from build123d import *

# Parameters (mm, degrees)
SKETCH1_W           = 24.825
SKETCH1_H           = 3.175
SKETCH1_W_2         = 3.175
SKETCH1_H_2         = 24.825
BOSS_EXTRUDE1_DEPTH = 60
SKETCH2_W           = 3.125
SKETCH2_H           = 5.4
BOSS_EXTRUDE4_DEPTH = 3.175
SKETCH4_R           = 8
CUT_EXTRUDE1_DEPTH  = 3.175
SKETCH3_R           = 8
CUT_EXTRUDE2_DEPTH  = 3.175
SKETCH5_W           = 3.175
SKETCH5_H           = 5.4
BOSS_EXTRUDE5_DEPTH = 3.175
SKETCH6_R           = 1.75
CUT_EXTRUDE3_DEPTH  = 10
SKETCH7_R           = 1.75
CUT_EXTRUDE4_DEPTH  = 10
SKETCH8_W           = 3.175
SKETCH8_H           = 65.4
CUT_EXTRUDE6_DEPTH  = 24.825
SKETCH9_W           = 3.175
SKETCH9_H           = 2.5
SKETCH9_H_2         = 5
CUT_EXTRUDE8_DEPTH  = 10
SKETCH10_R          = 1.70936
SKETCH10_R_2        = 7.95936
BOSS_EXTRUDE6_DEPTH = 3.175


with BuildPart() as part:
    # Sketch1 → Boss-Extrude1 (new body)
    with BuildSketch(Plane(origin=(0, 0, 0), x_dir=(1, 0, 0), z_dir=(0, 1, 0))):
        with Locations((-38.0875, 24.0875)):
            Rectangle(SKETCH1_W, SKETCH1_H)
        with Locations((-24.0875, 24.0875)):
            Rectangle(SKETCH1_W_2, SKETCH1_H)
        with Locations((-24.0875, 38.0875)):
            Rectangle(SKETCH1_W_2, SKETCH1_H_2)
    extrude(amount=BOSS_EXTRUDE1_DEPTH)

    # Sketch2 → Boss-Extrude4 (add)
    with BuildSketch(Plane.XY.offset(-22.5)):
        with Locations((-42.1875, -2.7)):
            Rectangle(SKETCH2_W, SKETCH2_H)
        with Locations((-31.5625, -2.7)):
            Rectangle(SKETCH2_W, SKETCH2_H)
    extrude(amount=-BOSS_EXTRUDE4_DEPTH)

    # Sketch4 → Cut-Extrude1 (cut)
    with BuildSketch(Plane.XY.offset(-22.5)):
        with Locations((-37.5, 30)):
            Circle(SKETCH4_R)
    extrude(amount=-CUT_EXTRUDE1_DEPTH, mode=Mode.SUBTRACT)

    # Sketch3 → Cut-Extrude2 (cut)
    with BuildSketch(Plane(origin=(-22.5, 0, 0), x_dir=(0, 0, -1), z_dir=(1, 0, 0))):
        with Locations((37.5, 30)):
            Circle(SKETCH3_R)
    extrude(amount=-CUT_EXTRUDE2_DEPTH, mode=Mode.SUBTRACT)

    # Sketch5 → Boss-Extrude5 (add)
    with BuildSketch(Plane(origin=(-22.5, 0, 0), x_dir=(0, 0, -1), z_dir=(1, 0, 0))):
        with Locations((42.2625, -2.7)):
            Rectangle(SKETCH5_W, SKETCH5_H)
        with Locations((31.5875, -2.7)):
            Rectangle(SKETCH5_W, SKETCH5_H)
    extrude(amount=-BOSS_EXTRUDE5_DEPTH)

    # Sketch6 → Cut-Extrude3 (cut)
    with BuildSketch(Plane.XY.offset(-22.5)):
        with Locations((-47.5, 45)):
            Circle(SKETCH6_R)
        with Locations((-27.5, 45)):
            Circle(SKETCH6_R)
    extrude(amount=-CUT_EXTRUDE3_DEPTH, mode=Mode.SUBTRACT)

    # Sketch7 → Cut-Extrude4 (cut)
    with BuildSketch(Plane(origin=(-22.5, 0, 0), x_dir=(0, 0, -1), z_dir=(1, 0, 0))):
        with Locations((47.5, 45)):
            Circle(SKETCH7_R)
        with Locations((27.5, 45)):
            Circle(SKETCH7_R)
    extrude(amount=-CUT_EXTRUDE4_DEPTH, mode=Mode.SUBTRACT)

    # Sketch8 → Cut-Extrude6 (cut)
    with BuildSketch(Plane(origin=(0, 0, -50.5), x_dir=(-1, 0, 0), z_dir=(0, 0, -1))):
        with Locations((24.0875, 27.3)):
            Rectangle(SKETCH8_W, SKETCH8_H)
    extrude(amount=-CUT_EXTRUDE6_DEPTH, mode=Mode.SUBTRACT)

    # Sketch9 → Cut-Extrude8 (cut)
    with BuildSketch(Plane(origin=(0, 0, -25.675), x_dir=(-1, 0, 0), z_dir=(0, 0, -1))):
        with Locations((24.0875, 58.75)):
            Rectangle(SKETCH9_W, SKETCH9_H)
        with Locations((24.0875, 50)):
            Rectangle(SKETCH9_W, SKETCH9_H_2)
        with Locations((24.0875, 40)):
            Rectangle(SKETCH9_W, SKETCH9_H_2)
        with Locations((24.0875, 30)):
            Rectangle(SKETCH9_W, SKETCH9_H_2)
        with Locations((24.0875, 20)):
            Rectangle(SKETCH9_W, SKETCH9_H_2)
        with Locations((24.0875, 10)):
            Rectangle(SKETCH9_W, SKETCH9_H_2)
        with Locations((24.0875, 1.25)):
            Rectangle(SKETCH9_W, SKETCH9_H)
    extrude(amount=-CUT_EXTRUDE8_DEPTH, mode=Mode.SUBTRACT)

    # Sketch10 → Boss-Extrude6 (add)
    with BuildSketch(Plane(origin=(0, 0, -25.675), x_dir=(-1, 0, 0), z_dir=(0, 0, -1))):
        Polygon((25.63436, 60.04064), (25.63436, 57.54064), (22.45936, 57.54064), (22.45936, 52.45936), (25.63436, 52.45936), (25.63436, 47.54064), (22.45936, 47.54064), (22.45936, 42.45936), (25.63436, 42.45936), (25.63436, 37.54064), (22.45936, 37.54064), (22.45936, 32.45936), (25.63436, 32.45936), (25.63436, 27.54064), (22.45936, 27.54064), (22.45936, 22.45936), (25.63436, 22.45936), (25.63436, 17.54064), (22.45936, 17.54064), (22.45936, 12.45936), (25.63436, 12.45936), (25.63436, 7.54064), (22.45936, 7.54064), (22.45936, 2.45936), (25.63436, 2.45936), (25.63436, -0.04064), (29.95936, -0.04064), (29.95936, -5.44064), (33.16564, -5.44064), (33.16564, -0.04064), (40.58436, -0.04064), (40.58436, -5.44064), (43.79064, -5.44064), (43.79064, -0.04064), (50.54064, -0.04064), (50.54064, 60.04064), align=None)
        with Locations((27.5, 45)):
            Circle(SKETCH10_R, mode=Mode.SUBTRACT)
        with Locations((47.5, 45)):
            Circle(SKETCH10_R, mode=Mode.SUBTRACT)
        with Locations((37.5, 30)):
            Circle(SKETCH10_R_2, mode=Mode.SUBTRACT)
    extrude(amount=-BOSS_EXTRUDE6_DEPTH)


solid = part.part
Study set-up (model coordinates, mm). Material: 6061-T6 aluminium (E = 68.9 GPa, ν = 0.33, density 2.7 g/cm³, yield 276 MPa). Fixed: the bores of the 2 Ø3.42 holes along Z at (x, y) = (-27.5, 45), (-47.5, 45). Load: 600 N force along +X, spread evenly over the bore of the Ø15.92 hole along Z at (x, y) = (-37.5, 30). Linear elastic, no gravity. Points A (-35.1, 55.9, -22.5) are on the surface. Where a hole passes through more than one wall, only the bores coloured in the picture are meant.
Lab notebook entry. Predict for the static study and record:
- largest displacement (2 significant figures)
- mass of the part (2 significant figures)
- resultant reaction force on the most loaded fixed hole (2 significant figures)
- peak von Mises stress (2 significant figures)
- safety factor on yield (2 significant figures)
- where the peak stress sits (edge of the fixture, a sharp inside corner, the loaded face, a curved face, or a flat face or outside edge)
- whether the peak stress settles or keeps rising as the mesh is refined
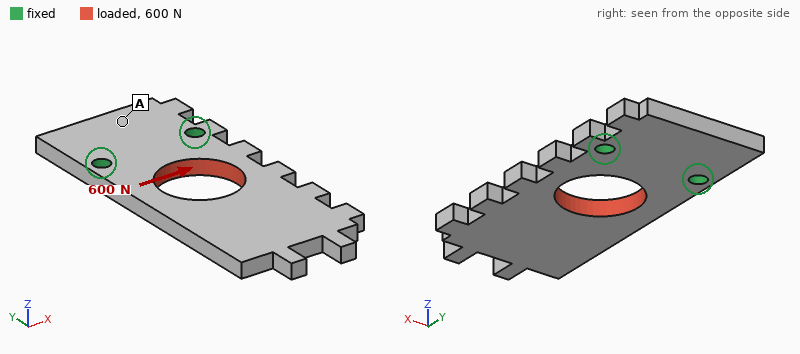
38 µm
12 g
500 N
66 MPa
4.2
the loaded face
settles
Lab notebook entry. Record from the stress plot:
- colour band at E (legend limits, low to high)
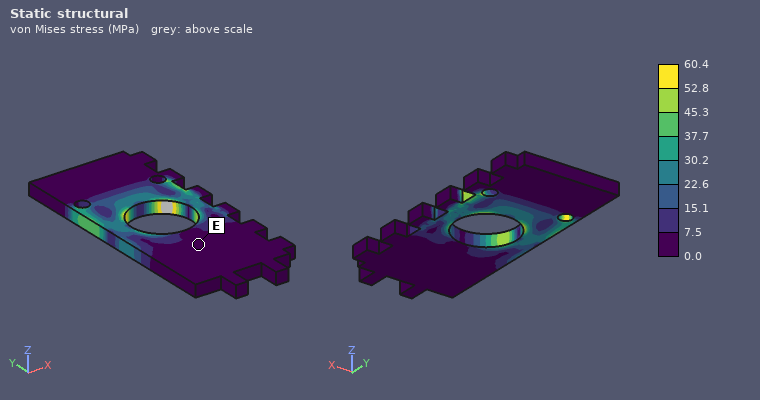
0.0 to 7.5 MPa
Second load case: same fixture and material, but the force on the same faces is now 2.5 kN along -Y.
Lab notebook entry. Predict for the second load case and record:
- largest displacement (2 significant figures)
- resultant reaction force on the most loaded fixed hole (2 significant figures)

18 µm
1.3 kN
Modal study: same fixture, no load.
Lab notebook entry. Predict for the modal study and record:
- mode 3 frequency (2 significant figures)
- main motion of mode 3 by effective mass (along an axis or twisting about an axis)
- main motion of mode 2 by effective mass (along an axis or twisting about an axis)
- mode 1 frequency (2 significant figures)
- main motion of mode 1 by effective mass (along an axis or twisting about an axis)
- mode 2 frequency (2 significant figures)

5600 Hz
along X
twisting about Y
910 Hz
along Z
3600 Hz
